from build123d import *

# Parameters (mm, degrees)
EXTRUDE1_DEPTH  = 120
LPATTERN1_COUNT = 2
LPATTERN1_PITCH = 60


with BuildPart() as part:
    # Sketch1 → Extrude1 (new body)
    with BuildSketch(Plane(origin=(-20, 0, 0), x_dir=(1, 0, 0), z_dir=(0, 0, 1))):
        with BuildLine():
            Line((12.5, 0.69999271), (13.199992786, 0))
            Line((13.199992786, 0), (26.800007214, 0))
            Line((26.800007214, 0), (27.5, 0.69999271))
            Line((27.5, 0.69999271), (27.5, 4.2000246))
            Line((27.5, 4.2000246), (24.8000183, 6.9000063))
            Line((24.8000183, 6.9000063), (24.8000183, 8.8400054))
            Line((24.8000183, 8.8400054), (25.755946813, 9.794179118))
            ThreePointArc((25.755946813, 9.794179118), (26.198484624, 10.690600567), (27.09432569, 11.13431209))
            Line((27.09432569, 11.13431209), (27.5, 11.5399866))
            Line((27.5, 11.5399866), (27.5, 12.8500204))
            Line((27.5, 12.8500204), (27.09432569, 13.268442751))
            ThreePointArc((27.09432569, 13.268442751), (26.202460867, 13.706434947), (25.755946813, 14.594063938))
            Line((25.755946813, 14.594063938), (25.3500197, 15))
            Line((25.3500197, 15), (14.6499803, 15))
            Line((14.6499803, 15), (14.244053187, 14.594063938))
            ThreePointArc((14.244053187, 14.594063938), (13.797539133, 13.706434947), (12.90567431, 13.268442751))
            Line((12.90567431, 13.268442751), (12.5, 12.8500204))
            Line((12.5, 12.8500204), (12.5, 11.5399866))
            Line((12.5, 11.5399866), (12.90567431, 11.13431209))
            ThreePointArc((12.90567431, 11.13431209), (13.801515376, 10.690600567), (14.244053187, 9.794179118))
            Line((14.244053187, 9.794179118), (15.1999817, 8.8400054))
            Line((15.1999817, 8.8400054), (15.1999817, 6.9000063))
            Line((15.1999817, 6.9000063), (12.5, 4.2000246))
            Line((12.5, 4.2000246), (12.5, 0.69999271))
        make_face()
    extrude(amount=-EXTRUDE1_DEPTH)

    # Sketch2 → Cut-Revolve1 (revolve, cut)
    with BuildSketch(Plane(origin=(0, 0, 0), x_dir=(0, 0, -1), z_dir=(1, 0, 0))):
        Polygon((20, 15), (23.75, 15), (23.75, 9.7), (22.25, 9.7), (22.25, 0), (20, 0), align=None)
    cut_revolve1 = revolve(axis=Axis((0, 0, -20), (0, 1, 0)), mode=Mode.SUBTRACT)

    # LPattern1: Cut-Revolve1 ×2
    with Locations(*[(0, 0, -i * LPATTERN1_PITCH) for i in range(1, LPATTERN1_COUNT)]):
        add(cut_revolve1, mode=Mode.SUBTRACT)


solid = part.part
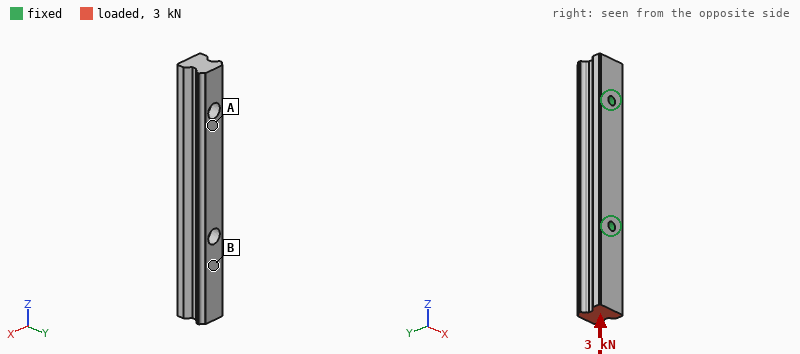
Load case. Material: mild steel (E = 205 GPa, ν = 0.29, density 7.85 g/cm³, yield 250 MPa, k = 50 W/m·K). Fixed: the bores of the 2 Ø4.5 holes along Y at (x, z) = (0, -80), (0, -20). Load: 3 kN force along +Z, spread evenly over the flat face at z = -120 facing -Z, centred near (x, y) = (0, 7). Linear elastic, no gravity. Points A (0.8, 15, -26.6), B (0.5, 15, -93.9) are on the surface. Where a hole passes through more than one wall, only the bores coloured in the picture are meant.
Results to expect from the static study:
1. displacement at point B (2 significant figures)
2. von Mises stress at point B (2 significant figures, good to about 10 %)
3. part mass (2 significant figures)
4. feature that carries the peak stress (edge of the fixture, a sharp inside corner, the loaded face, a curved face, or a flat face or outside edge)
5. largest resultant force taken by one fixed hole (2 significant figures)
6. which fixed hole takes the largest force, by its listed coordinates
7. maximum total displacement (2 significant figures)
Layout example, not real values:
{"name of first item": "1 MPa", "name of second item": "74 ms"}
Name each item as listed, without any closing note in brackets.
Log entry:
{"displacement at point B": "2.6 µm", "von Mises stress at point B": "14 MPa", "part mass": "180 g", "feature that carries the peak stress": "edge of the fixture", "largest resultant force taken by one fixed hole": "2.8 kN", "which fixed hole takes the largest force, by its listed coordinates": "(0, -80)", "maximum total displacement": "5.8 µm"}
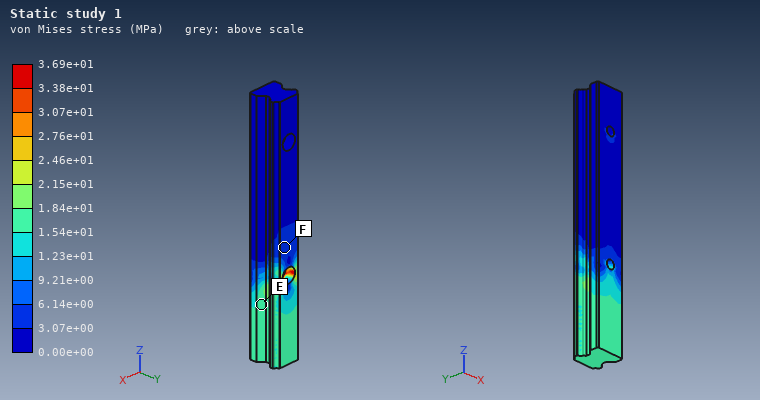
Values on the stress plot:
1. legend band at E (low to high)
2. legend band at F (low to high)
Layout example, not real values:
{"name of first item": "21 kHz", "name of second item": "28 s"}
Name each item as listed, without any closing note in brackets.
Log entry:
{"legend band at E": "1.54e+01 to 1.84e+01 MPa", "legend band at F": "3.07e+00 to 6.14e+00 MPa"}
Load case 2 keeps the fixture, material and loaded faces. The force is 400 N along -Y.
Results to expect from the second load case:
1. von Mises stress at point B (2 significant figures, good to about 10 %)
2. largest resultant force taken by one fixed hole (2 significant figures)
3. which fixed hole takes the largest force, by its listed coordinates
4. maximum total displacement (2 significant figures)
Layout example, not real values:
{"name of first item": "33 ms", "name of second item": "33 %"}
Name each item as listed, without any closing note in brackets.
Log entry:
{"von Mises stress at point B": "20 MPa", "largest resultant force taken by one fixed hole": "520 N", "which fixed hole takes the largest force, by its listed coordinates": "(0, -80)", "maximum total displacement": "18 µm"}
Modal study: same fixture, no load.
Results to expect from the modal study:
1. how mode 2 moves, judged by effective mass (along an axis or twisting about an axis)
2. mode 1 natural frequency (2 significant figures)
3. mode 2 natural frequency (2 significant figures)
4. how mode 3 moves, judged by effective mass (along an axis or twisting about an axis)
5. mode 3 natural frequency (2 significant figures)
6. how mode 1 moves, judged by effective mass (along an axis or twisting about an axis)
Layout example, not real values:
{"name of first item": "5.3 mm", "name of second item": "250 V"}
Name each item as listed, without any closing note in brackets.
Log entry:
{"how mode 2 moves, judged by effective mass": "along Y", "mode 1 natural frequency": "5100 Hz", "mode 2 natural frequency": "5700 Hz", "how mode 3 moves, judged by effective mass": "along X", "mode 3 natural frequency": "12 kHz", "how mode 1 moves, judged by effective mass": "along X"}
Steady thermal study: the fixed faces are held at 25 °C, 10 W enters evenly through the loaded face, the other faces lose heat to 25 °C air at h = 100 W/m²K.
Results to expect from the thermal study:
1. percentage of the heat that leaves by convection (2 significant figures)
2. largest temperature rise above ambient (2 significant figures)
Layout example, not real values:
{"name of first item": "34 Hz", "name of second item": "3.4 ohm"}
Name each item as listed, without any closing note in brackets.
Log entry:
{"percentage of the heat that leaves by convection": "39 %", "largest temperature rise above ambient": "32 K"}
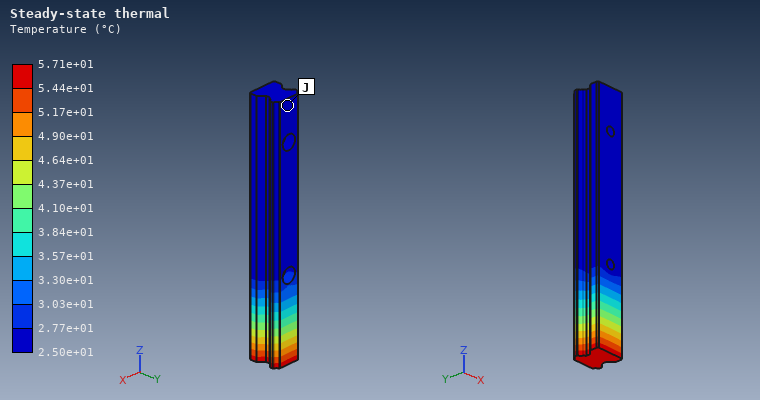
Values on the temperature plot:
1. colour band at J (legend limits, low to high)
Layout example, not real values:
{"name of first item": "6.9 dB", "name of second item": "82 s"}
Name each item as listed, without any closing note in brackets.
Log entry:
{"colour band at J": "2.50e+01 to 2.77e+01 °C"}
